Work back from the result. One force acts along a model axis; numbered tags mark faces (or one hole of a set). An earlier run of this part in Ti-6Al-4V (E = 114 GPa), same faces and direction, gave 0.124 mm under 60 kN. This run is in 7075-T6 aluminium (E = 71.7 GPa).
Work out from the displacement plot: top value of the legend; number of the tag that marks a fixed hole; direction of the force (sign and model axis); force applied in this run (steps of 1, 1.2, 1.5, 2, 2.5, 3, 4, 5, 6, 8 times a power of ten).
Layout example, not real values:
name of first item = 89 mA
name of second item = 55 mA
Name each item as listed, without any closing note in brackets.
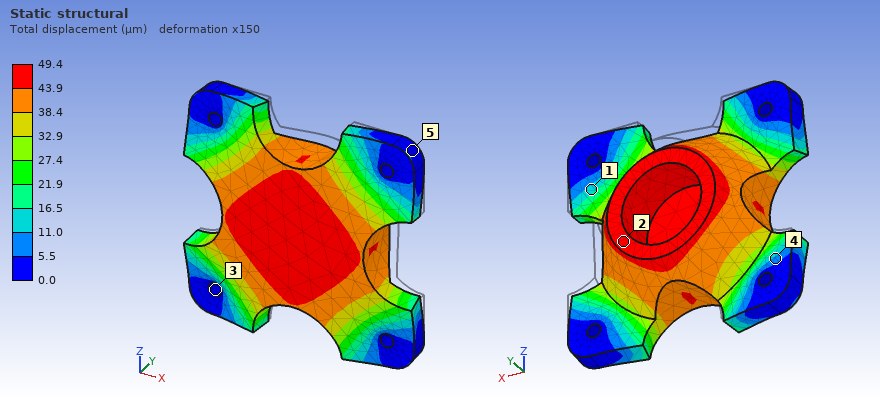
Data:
top value of the legend = 49.4 µm
number of the tag that marks a fixed hole = 3
direction of the force = -Y
force applied in this run = 15 kN
